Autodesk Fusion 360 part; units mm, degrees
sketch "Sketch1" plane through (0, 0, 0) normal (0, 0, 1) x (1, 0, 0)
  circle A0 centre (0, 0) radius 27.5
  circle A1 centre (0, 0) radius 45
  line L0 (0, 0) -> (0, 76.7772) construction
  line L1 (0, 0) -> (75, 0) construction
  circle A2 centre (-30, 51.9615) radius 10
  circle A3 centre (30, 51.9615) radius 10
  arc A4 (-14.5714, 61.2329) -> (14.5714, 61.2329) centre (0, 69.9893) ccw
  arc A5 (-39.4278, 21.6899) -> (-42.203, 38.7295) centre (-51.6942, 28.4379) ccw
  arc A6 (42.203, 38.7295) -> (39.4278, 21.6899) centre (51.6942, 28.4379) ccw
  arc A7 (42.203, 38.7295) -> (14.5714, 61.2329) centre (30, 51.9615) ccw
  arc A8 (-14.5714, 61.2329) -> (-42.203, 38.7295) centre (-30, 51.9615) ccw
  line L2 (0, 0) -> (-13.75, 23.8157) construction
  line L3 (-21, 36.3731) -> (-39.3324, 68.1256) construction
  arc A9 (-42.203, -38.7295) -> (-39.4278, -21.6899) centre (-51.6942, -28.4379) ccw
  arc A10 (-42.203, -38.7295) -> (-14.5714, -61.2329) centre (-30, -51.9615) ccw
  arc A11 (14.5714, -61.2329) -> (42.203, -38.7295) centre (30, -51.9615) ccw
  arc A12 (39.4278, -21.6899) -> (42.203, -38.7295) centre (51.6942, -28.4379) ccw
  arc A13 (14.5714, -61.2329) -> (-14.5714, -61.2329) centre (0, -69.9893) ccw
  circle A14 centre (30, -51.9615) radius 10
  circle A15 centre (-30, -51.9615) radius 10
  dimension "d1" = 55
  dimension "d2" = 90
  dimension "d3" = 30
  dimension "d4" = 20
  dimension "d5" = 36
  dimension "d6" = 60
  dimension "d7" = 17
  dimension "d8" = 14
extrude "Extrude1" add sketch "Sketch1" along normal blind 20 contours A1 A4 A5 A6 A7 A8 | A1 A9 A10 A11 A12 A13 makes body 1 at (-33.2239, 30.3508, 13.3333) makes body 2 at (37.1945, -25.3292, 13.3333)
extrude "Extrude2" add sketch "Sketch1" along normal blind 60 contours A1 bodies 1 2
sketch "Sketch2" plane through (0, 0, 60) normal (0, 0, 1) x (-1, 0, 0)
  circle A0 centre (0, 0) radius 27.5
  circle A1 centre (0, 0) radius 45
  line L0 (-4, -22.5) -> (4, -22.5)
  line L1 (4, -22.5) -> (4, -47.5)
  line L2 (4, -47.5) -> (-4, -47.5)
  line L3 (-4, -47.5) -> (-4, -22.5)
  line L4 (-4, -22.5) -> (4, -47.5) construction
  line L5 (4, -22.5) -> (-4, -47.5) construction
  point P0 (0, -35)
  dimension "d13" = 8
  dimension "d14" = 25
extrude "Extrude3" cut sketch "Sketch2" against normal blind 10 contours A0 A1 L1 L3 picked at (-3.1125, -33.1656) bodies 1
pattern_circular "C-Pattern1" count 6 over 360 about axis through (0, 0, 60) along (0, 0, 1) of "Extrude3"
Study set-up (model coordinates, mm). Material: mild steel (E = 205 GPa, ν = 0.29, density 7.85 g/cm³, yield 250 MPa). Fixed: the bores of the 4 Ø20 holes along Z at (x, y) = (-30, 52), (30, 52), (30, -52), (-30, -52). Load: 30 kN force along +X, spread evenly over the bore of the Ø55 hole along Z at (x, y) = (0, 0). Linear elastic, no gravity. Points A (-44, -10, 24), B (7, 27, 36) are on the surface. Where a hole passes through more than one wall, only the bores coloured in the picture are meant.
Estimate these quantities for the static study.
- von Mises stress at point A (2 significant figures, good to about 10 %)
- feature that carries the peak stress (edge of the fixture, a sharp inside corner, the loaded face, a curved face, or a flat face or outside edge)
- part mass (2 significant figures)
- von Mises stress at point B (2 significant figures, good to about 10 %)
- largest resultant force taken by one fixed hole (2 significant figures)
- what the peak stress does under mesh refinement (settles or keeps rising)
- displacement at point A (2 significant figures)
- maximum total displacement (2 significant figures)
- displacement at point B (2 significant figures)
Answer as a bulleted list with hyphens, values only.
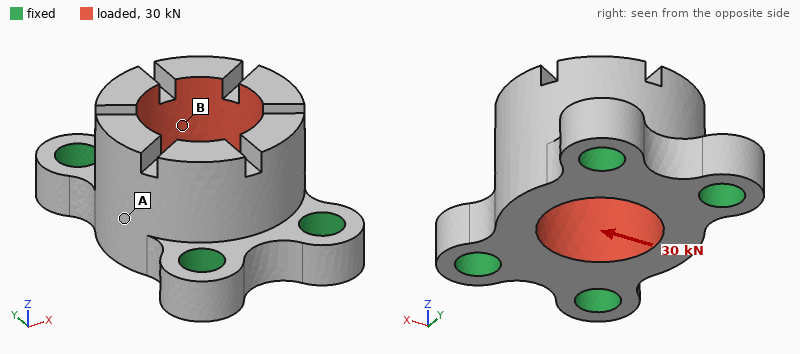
- 6.9 MPa
- edge of the fixture
- 2.3 kg
- 18 MPa
- 9.4 kN
- keeps rising
- 6.6 µm
- 12 µm
- 5.4 µm
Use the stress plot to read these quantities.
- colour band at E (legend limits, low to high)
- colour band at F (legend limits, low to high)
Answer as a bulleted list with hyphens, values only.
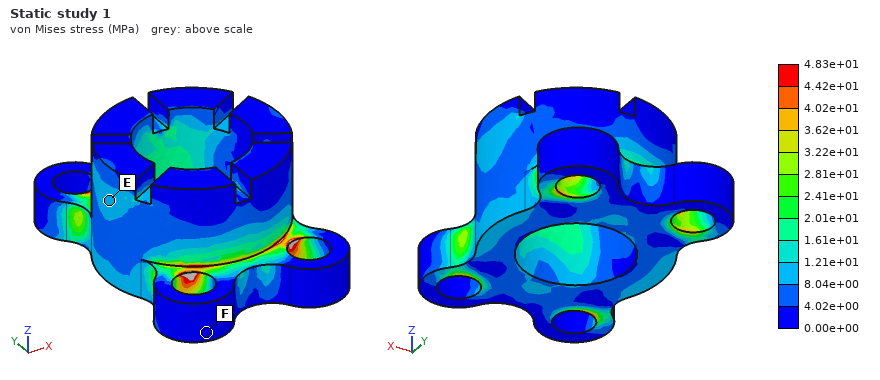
- 8.04e+00 to 1.21e+01 MPa
- 0.00e+00 to 4.02e+00 MPa
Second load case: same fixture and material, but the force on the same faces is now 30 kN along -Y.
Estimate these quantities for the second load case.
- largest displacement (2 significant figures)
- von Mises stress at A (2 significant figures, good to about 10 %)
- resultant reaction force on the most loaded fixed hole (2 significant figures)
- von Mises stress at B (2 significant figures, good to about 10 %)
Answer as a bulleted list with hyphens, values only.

- 6.8 µm
- 4.7 MPa
- 8.3 kN
- 5.4 MPa
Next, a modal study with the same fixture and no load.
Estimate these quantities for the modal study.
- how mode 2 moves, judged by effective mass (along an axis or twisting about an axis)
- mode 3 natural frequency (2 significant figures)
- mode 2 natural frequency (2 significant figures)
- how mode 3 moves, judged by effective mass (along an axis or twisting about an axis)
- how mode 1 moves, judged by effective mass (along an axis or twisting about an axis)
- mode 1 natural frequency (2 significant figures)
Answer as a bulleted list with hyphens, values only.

- along Z
- 10 kHz
- 7900 Hz
- along Y
- along X
- 6800 Hz
